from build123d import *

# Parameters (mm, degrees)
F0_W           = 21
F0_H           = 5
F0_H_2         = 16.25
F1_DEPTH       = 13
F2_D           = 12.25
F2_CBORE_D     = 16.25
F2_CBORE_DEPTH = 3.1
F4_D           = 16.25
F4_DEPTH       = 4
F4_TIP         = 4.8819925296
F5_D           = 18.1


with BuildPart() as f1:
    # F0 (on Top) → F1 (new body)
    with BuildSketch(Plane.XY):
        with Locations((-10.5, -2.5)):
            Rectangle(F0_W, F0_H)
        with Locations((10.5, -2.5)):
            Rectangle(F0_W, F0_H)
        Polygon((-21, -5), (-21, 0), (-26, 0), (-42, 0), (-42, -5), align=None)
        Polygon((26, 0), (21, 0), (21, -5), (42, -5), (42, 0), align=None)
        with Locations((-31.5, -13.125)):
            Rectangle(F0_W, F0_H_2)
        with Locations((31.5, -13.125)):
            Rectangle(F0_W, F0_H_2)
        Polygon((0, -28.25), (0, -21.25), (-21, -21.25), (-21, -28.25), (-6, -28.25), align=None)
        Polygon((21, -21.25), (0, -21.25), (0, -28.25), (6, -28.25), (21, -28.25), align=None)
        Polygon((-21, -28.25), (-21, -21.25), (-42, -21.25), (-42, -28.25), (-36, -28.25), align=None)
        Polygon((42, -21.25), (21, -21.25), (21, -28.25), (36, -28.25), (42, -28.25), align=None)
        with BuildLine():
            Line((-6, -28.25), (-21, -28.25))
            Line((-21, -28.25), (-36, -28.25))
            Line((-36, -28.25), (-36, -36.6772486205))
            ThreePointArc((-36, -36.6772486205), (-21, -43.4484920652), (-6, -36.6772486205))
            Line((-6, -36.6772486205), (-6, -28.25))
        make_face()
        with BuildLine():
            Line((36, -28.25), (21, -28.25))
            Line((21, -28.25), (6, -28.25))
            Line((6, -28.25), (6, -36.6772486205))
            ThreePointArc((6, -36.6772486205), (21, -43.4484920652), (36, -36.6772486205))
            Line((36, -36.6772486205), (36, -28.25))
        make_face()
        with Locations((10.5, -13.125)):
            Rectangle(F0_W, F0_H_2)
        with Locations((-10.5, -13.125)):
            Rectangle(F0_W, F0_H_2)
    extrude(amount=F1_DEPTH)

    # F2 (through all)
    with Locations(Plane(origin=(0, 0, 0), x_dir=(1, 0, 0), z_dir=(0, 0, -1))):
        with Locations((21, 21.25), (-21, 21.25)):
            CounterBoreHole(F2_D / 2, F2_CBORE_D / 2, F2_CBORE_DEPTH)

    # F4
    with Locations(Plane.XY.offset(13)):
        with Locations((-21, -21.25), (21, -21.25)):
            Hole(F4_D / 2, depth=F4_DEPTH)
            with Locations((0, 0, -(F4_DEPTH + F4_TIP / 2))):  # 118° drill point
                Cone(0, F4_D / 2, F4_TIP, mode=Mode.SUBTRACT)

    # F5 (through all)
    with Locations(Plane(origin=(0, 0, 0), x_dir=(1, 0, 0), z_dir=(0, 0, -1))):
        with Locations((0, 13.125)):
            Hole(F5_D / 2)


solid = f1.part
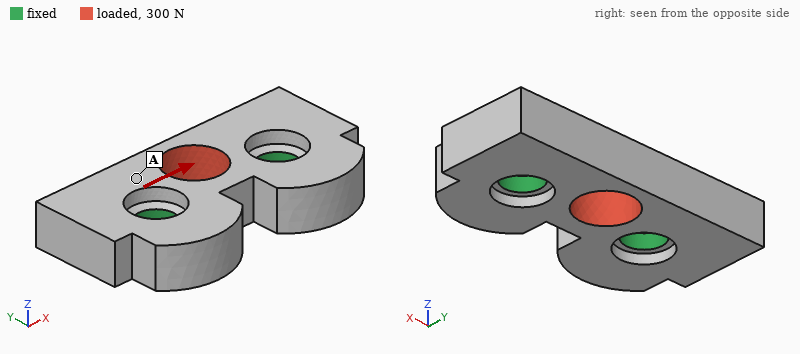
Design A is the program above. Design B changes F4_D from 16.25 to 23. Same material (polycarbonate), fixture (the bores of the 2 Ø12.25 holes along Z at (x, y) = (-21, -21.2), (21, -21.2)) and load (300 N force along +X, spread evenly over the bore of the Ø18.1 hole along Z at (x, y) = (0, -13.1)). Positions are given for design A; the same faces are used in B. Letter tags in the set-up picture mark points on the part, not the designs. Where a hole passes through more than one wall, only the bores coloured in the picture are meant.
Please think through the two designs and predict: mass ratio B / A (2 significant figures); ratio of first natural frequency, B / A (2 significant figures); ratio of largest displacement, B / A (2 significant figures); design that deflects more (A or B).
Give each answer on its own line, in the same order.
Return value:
0.93
0.80
1.2
B
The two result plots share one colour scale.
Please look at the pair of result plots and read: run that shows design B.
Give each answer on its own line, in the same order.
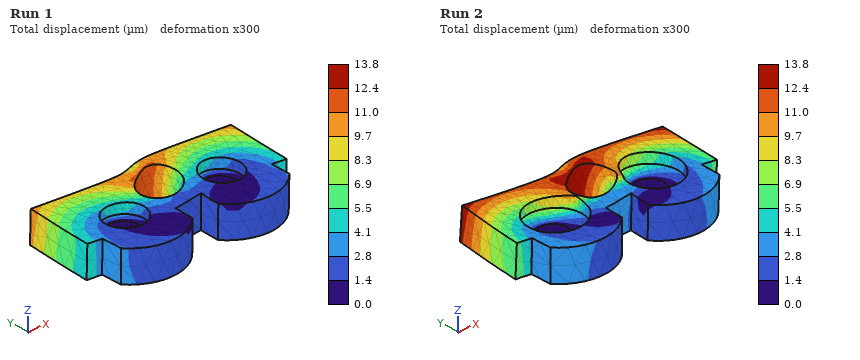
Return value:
Run 2
